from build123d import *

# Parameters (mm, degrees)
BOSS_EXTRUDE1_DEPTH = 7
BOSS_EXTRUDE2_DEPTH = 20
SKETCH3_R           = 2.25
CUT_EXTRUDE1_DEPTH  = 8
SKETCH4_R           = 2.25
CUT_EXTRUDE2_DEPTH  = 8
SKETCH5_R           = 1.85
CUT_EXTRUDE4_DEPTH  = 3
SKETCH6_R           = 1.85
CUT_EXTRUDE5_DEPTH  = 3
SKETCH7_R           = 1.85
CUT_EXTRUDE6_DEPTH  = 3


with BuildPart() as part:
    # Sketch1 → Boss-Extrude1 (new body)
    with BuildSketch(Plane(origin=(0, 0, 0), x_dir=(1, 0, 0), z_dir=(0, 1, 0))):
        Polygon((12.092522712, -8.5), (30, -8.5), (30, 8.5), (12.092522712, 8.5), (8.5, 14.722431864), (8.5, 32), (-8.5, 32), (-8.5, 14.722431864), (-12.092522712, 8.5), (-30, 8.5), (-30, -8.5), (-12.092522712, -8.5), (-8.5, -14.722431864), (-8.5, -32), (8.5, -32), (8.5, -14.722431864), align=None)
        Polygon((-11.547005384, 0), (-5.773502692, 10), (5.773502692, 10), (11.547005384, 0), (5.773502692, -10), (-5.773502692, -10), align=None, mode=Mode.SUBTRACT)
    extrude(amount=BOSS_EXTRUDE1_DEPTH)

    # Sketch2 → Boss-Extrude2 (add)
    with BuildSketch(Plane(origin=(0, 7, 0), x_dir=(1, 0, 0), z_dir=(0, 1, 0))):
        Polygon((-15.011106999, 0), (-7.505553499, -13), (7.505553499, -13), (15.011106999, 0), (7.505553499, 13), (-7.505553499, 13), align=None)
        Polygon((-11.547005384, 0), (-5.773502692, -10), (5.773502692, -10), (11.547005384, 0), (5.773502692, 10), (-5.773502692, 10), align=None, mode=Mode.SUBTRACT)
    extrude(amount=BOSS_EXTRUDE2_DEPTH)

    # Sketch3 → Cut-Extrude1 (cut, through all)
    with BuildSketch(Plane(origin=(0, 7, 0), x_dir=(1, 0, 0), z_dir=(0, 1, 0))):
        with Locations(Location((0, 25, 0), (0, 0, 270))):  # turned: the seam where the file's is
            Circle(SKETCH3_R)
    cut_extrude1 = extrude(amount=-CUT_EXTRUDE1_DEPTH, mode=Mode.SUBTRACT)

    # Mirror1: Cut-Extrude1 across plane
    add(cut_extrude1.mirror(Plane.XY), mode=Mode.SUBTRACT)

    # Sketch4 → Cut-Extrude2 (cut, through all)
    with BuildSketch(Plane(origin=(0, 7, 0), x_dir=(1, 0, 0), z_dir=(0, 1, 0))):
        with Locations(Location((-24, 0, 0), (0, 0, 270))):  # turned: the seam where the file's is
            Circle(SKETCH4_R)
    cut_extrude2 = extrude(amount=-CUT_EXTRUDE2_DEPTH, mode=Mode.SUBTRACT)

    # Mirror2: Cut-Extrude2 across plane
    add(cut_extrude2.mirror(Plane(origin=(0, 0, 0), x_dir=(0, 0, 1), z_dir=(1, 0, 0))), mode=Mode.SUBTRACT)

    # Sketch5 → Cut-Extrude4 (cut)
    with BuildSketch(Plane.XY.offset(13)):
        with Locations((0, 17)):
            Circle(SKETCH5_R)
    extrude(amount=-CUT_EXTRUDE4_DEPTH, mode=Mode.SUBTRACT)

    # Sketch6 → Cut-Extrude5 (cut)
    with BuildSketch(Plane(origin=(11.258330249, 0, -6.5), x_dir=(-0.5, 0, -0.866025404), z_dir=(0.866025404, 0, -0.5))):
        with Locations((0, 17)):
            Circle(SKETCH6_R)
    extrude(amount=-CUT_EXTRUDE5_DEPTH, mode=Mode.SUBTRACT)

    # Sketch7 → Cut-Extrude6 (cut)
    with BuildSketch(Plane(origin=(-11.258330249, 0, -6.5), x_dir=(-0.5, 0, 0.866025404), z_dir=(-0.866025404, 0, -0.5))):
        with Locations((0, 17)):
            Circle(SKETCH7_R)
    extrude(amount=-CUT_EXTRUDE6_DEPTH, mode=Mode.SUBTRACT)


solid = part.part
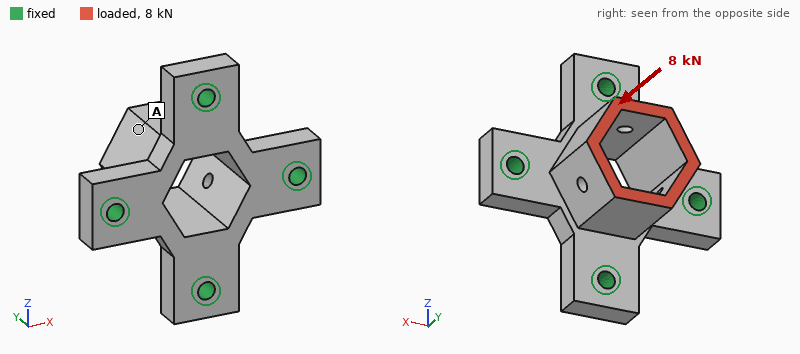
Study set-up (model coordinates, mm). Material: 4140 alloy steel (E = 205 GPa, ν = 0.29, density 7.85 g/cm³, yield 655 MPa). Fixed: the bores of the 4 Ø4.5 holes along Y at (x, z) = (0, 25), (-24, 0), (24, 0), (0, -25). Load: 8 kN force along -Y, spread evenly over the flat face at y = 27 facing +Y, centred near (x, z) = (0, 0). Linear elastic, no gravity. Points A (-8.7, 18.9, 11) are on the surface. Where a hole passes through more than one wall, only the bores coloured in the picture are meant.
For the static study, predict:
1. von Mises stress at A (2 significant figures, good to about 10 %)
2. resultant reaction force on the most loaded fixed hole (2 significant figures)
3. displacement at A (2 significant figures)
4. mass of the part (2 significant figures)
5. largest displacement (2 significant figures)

28 MPa
2.2 kN
12 µm
120 g
14 µm
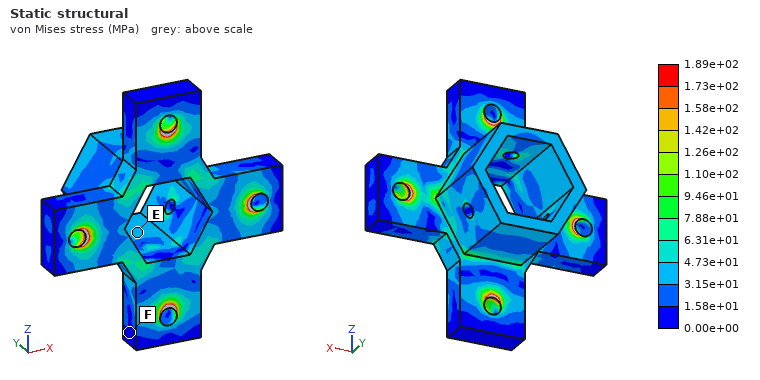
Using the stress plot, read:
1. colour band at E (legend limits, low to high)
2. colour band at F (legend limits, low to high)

3.15e+01 to 4.73e+01 MPa
0.00e+00 to 1.58e+01 MPa
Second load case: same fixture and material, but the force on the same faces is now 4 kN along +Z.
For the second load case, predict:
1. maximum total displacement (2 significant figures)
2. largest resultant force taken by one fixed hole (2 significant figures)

38 µm
2.8 kN
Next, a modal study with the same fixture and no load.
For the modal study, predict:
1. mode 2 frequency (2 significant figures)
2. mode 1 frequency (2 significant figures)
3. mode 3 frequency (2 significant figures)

15 kHz
14 kHz
17 kHz
